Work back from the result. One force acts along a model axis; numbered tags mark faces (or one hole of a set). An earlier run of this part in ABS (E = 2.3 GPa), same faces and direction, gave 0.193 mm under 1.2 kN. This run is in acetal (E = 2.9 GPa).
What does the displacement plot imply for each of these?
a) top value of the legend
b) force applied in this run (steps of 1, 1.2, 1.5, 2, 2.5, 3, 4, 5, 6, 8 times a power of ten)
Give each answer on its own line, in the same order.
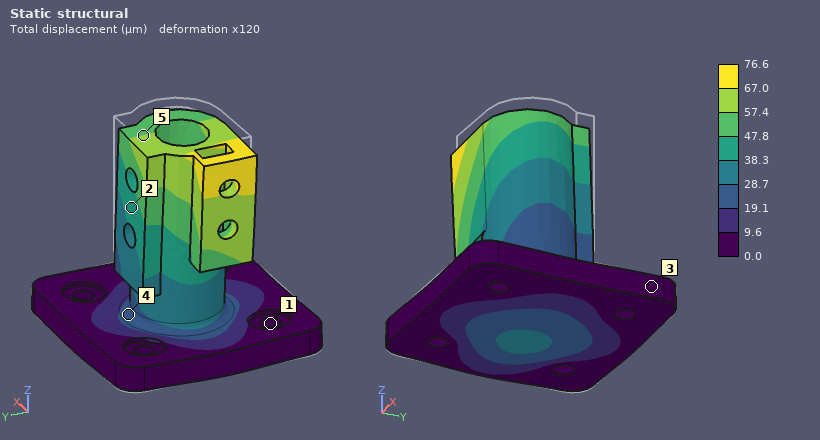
76.6 µm
600 N
